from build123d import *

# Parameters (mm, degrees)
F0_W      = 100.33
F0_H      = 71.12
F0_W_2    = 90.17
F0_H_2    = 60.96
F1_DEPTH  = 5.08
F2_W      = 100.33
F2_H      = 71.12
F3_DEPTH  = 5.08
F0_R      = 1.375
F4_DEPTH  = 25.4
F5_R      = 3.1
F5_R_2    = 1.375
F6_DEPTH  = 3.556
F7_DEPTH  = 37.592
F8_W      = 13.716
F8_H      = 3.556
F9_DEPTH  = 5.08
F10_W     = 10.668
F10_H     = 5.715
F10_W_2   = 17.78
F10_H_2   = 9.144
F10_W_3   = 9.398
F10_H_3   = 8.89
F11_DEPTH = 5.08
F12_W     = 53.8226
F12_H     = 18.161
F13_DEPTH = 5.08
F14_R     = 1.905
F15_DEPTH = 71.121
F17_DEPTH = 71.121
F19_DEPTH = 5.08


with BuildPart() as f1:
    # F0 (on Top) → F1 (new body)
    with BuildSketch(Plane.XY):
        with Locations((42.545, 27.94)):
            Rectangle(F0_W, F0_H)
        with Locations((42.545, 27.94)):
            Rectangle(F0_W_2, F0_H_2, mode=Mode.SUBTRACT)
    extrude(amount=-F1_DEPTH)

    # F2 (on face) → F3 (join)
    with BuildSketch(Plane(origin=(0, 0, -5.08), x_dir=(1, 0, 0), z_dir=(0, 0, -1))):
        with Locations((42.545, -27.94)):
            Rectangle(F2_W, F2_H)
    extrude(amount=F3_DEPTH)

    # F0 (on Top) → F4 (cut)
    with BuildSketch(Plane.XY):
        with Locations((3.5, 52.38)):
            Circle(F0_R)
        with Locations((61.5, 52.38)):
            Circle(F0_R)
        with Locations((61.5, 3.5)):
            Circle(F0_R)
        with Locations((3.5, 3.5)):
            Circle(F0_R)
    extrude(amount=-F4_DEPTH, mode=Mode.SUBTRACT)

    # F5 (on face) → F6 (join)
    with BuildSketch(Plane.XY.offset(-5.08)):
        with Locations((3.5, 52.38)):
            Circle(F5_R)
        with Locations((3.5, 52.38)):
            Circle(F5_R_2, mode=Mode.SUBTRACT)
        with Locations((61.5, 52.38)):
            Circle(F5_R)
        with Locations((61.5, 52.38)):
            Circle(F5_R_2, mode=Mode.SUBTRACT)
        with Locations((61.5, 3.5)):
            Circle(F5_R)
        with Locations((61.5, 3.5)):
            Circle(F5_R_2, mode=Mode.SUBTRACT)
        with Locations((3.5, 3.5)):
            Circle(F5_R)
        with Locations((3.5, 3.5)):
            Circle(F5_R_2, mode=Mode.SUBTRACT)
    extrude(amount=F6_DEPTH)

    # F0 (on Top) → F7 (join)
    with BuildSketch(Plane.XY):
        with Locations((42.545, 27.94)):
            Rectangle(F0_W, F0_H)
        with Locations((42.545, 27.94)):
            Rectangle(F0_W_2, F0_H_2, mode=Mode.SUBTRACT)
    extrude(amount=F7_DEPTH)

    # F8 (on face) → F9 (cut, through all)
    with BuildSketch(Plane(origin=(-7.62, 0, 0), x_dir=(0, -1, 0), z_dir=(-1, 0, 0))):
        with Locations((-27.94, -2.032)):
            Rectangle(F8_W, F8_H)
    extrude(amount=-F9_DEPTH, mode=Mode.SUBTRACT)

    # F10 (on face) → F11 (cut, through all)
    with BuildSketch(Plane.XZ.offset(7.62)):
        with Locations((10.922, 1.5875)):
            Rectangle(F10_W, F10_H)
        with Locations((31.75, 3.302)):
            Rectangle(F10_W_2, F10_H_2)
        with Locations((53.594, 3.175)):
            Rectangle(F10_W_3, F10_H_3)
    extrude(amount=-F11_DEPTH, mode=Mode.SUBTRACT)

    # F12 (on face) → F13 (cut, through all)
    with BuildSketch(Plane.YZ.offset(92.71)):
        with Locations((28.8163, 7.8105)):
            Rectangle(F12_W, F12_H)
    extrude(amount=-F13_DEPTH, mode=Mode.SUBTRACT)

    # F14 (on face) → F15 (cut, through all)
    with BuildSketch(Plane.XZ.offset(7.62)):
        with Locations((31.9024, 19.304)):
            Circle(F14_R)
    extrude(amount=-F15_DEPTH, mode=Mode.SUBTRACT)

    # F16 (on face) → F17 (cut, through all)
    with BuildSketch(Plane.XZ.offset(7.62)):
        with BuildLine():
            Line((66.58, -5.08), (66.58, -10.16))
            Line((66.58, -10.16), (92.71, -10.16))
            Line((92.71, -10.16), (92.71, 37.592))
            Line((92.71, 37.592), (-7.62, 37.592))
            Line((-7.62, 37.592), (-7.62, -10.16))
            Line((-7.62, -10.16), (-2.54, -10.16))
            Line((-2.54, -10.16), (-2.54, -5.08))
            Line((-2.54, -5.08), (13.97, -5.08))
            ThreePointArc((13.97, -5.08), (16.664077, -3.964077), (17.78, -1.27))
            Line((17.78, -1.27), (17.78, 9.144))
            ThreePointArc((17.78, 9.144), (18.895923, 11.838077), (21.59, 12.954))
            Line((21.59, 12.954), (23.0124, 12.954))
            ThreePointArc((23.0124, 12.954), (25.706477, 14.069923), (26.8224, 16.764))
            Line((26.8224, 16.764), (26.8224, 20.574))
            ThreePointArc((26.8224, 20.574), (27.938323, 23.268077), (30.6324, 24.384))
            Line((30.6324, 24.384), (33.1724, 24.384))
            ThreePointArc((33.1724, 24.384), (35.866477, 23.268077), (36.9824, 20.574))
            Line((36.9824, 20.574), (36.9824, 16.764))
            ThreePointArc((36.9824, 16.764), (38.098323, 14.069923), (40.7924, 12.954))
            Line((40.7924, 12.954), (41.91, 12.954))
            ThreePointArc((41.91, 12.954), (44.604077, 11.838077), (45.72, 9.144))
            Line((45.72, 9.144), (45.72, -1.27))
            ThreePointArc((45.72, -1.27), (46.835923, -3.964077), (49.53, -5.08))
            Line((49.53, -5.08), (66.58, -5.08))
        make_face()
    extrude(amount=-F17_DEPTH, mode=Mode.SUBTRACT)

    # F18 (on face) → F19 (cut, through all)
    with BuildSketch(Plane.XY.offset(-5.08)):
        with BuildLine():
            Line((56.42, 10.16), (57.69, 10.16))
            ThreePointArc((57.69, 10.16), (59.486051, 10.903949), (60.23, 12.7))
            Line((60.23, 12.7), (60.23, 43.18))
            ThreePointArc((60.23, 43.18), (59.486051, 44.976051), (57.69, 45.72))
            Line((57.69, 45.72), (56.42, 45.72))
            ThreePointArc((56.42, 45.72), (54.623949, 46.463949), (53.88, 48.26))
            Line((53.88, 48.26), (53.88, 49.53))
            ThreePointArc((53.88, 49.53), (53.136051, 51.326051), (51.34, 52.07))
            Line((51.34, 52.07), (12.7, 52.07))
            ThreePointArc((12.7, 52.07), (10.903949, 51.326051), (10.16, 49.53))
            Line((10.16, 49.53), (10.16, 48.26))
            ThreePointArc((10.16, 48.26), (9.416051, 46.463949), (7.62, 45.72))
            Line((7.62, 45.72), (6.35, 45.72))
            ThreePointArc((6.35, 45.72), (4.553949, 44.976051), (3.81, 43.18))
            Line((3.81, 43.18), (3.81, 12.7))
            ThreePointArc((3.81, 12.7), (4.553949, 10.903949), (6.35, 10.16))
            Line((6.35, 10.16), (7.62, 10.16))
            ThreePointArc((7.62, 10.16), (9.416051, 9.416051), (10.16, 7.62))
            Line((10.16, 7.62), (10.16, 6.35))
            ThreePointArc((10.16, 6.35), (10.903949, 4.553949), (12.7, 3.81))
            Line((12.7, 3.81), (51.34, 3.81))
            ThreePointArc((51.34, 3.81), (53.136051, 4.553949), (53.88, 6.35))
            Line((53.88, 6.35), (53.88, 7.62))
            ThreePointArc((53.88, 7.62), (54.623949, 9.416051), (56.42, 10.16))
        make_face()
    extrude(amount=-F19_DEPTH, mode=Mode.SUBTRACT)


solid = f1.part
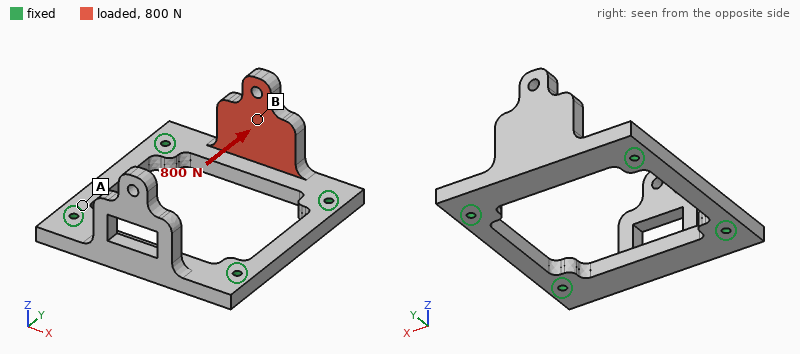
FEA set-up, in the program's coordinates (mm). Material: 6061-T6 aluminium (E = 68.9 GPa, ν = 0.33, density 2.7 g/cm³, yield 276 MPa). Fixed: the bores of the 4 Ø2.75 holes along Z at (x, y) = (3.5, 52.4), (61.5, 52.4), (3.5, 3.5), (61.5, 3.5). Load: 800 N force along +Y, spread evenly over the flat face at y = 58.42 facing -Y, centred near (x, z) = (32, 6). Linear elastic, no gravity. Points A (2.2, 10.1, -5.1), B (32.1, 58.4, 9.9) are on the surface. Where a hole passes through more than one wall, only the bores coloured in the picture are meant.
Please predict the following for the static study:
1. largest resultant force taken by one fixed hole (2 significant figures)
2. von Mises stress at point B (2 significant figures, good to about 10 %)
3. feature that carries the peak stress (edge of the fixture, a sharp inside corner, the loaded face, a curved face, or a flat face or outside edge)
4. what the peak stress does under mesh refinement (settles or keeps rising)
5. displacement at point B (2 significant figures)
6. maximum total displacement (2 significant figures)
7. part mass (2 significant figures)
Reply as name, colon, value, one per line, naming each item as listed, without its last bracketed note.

largest resultant force taken by one fixed hole: 670 N
von Mises stress at point B: 29 MPa
feature that carries the peak stress: edge of the fixture
what the peak stress does under mesh refinement: keeps rising
displacement at point B: 0.24 mm
maximum total displacement: 0.46 mm
part mass: 47 g
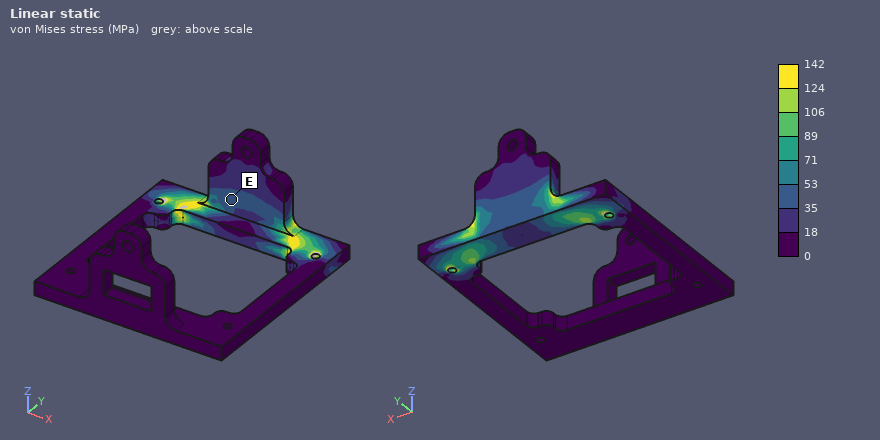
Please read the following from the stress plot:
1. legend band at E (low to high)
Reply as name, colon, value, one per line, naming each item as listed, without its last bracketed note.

legend band at E: 35 to 53 MPa
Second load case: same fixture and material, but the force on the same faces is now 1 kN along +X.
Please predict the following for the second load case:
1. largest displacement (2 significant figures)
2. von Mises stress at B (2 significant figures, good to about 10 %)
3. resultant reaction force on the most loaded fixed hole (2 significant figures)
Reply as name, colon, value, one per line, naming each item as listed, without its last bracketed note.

largest displacement: 58 µm
von Mises stress at B: 15 MPa
resultant reaction force on the most loaded fixed hole: 600 N
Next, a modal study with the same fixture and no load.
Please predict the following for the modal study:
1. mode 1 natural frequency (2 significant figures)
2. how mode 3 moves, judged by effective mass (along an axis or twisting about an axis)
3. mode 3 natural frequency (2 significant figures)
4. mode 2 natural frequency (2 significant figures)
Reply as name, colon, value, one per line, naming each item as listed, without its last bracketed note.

mode 1 natural frequency: 2900 Hz
how mode 3 moves, judged by effective mass: along Z
mode 3 natural frequency: 6400 Hz
mode 2 natural frequency: 3000 Hz
